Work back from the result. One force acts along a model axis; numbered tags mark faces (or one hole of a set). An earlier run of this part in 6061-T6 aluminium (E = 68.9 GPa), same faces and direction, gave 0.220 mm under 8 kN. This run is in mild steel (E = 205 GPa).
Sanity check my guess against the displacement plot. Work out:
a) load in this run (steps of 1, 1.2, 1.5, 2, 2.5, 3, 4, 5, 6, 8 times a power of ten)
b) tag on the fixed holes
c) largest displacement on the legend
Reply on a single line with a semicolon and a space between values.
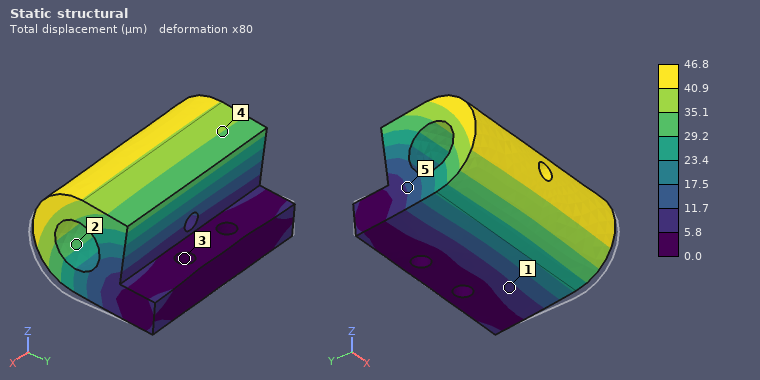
5 kN; 3; 46.8 µm
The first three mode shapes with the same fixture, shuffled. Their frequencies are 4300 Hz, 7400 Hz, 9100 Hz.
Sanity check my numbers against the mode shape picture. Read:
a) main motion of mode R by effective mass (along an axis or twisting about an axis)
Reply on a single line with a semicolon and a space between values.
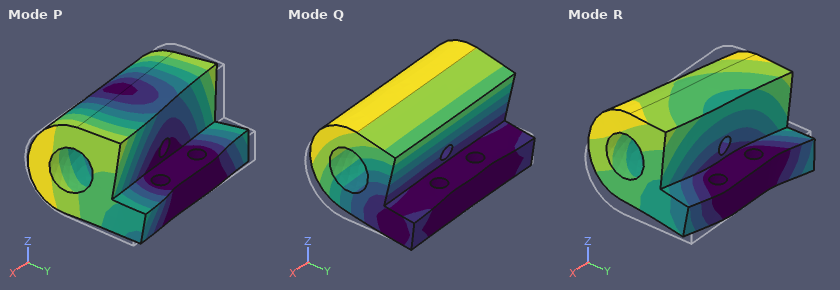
along X
